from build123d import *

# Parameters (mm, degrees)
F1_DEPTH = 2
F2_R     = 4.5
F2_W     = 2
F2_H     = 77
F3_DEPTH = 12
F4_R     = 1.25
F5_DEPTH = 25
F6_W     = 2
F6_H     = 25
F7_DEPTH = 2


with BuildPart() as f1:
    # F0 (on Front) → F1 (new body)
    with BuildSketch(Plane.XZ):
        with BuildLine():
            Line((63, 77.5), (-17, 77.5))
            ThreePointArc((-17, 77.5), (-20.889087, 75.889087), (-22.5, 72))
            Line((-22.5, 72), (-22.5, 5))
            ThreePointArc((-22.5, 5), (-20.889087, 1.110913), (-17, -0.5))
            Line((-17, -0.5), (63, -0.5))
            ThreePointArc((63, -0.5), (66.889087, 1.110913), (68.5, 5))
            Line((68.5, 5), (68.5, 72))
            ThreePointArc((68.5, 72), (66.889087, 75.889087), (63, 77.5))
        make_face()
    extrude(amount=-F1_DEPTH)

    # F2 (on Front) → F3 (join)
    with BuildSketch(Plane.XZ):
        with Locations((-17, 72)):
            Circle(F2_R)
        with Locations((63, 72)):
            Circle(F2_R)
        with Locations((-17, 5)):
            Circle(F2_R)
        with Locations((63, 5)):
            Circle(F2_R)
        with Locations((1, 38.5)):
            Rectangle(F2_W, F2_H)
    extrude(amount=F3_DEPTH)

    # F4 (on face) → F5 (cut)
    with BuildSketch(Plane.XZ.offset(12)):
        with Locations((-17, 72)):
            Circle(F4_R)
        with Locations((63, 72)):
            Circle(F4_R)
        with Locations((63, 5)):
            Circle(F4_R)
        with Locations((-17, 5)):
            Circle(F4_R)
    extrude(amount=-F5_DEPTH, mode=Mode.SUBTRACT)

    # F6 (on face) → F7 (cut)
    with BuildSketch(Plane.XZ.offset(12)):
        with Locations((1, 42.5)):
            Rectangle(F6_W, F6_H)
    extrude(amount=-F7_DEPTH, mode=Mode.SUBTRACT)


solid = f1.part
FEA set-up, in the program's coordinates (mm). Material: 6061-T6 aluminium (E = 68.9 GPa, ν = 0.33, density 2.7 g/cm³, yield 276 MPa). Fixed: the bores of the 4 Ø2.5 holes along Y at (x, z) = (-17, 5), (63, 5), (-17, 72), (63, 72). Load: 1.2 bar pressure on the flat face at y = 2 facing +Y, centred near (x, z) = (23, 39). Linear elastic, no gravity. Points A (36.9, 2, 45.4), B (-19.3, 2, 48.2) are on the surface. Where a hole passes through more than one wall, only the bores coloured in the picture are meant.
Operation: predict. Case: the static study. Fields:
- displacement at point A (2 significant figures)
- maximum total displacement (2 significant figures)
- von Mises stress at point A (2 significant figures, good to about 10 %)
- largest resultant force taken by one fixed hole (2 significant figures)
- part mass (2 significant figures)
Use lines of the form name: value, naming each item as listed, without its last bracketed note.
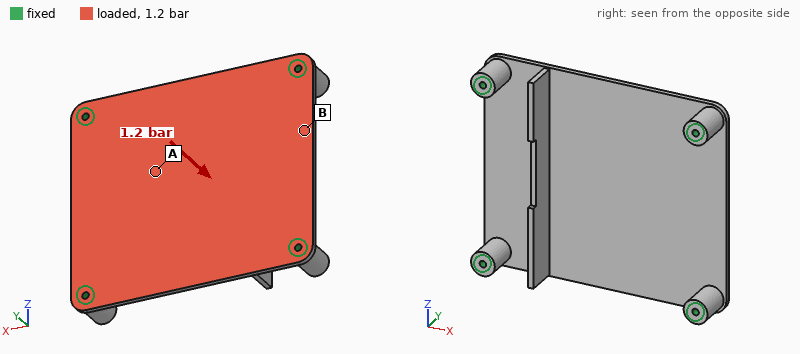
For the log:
displacement at point A: 0.33 mm
maximum total displacement: 0.36 mm
von Mises stress at point A: 38 MPa
largest resultant force taken by one fixed hole: 230 N
part mass: 50 g
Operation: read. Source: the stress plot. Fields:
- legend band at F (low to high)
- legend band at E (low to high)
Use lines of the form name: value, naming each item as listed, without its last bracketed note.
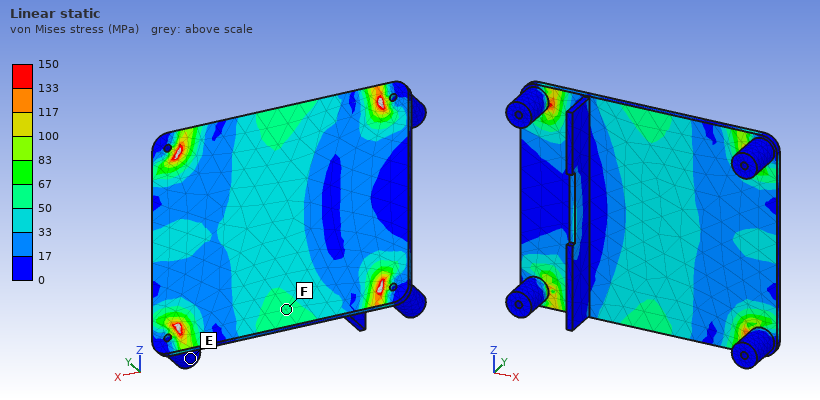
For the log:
legend band at F: 50 to 67 MPa
legend band at E: 0 to 17 MPa
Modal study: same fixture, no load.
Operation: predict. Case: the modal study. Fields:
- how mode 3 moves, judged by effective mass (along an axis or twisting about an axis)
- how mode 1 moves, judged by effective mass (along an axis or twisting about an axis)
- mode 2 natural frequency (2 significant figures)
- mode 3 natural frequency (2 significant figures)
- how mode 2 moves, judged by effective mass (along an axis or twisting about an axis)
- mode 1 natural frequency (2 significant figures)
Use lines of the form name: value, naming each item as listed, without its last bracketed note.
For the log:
how mode 3 moves, judged by effective mass: twisting about Z
how mode 1 moves, judged by effective mass: along Y
mode 2 natural frequency: 2100 Hz
mode 3 natural frequency: 2700 Hz
how mode 2 moves, judged by effective mass: twisting about X
mode 1 natural frequency: 1400 Hz
